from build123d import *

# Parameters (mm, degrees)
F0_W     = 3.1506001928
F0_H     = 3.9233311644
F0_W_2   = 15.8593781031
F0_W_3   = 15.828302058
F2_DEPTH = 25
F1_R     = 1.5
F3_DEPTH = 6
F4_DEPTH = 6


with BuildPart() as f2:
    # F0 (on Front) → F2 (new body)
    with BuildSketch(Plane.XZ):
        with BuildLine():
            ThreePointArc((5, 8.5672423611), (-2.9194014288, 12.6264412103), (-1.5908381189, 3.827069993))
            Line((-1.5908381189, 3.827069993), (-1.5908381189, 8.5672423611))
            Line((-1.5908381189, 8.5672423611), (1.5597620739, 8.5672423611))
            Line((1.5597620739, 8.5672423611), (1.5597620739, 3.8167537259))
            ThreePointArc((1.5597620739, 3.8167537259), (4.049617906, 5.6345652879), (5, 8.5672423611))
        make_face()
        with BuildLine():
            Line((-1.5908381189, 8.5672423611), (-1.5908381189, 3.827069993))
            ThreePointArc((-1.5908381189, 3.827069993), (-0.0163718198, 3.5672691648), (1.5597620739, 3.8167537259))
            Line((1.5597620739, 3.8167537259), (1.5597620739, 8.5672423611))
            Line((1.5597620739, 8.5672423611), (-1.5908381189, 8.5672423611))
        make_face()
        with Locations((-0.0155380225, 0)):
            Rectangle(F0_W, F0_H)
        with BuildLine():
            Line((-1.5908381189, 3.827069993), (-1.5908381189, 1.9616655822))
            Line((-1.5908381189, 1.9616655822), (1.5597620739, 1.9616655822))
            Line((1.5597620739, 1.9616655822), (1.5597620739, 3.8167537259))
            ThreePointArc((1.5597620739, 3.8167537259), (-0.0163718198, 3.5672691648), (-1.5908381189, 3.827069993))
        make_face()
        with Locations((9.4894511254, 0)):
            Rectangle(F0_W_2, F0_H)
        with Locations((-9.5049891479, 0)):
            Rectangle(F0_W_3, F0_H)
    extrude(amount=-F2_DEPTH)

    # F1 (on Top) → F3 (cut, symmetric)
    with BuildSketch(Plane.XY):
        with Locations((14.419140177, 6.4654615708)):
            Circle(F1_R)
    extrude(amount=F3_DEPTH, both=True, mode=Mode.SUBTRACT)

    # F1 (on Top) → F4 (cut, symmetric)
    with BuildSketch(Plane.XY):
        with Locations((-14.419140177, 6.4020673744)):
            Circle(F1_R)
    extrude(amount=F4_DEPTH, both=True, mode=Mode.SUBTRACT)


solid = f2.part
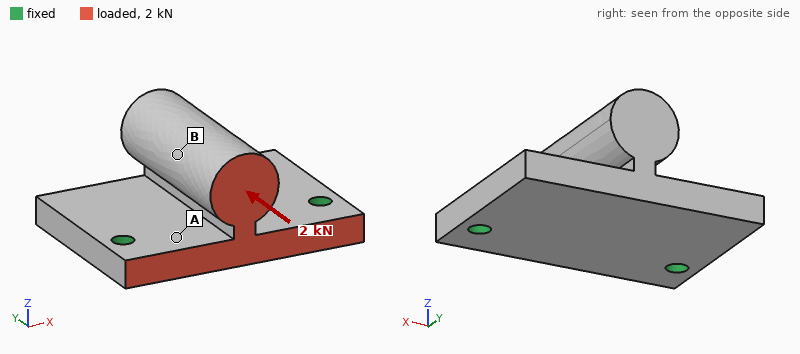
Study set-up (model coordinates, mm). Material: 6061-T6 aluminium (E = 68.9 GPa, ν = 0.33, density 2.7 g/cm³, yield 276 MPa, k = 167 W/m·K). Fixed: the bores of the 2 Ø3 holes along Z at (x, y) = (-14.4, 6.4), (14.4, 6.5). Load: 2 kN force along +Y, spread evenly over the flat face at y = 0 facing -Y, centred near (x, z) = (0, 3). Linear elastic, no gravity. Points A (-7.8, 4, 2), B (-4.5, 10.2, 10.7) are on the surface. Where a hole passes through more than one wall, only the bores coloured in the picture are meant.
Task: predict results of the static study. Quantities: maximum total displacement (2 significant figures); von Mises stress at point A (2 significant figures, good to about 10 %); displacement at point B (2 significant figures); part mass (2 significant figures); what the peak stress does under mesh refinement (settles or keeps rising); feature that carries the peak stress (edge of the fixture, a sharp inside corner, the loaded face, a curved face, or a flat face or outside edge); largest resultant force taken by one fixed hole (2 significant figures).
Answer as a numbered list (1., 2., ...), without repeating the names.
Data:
1. 0.10 mm
2. 60 MPa
3. 0.055 mm
4. 15 g
5. keeps rising
6. edge of the fixture
7. 1.0 kN
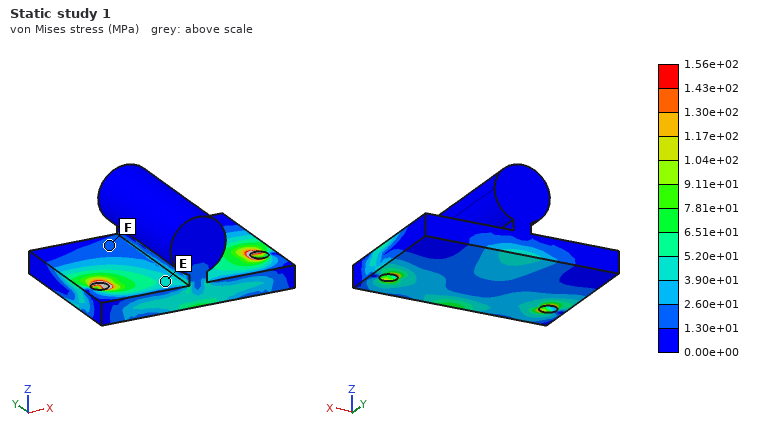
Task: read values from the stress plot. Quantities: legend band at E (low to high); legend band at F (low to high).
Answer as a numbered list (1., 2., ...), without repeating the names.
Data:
1. 3.90e+01 to 5.20e+01 MPa
2. 1.30e+01 to 2.60e+01 MPa
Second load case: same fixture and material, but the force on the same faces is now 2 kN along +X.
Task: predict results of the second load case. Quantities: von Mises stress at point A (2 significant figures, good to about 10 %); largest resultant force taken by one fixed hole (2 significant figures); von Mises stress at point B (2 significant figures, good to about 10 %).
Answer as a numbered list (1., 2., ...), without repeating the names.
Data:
1. 41 MPa
2. 1.1 kN
3. 27 MPa
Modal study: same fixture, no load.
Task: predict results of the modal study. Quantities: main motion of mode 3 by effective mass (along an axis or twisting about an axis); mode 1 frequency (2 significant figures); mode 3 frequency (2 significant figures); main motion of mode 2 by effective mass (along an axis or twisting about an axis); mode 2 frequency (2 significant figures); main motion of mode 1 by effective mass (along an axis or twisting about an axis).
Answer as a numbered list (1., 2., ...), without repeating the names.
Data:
1. along Z
2. 5000 Hz
3. 12 kHz
4. along X
5. 8600 Hz
6. along Z
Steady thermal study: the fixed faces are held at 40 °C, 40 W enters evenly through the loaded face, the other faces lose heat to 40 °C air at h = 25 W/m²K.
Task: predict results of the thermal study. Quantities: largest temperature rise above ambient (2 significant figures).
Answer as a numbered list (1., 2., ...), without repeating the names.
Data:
1. 30 K
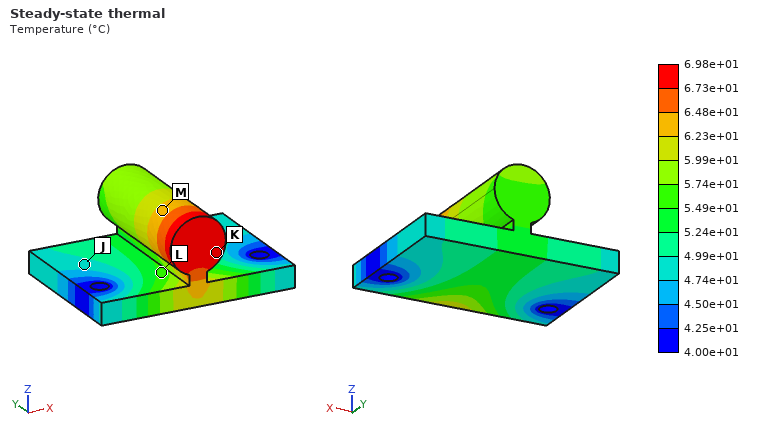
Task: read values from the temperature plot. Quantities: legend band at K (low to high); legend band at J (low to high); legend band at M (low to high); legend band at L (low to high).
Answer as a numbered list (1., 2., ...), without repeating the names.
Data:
1. 6.73e+01 to 6.98e+01 °C
2. 4.74e+01 to 4.99e+01 °C
3. 6.23e+01 to 6.48e+01 °C
4. 5.49e+01 to 5.74e+01 °C
